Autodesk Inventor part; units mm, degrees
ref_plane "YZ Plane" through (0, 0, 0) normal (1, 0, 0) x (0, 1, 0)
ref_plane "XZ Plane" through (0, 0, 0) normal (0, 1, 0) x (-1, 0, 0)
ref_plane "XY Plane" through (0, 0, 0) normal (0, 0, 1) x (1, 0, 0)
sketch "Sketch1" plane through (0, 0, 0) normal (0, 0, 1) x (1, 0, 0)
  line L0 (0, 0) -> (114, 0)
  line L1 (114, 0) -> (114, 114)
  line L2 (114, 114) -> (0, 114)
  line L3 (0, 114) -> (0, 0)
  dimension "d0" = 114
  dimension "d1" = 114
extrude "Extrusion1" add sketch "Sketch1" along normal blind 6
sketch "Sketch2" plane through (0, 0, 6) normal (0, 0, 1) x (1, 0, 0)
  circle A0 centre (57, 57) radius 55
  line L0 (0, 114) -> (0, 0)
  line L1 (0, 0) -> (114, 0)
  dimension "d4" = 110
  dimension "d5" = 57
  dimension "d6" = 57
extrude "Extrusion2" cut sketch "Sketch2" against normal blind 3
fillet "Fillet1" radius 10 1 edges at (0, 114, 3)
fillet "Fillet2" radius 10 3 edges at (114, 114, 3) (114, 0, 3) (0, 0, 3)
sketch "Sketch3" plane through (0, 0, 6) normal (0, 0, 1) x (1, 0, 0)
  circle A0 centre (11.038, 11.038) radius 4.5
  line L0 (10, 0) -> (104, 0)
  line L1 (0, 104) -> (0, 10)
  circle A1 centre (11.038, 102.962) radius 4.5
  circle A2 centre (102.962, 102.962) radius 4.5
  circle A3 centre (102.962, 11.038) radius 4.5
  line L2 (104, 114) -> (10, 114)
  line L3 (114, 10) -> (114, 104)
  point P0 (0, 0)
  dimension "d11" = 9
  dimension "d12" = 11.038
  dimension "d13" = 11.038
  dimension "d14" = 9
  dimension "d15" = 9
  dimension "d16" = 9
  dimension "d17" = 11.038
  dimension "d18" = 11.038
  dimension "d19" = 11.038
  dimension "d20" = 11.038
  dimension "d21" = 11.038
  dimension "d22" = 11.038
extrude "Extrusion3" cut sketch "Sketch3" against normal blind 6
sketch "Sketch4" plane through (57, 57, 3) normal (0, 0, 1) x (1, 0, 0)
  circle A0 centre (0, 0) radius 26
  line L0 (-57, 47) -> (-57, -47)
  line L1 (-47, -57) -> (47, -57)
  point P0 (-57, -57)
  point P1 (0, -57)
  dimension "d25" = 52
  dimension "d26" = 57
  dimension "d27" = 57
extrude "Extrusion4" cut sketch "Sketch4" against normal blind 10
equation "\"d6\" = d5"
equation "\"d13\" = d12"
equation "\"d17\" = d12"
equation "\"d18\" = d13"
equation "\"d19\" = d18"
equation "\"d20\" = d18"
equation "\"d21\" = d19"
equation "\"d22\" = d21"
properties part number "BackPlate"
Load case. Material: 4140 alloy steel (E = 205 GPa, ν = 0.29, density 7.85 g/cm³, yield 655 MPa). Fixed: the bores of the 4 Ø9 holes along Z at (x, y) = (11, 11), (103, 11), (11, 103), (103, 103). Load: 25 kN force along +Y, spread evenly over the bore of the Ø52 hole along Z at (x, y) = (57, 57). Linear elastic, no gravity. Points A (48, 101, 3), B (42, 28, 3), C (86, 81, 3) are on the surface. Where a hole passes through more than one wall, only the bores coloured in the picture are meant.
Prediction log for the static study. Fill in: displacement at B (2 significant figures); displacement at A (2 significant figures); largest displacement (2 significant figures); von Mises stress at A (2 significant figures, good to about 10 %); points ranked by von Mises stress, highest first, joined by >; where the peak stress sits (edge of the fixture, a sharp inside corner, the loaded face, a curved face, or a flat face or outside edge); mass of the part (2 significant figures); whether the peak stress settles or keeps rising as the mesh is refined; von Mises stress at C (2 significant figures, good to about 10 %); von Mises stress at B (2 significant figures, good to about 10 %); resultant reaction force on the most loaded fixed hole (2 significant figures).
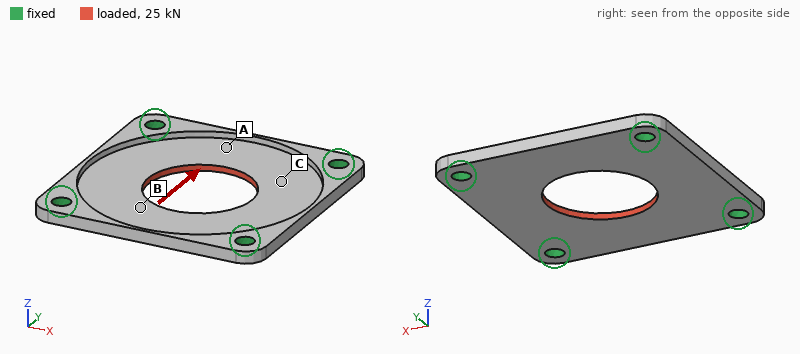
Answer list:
21 µm
21 µm
28 µm
37 MPa
C > B > A
edge of the fixture
320 g
keeps rising
66 MPa
55 MPa
6.6 kN
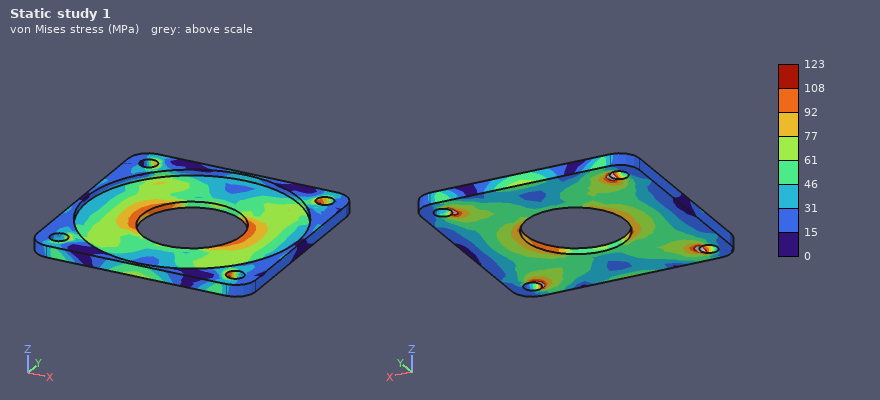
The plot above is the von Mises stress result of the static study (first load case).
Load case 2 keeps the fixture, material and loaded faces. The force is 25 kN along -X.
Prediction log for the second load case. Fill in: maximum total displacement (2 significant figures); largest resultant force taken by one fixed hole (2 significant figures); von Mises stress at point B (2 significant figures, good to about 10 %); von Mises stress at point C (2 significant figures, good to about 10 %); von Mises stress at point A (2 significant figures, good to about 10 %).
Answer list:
28 µm
6.6 kN
82 MPa
61 MPa
52 MPa
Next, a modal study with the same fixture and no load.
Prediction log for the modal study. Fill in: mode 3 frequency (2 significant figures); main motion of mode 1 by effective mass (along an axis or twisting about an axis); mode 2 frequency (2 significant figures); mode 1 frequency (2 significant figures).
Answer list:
3400 Hz
along Z
3400 Hz
2600 Hz
